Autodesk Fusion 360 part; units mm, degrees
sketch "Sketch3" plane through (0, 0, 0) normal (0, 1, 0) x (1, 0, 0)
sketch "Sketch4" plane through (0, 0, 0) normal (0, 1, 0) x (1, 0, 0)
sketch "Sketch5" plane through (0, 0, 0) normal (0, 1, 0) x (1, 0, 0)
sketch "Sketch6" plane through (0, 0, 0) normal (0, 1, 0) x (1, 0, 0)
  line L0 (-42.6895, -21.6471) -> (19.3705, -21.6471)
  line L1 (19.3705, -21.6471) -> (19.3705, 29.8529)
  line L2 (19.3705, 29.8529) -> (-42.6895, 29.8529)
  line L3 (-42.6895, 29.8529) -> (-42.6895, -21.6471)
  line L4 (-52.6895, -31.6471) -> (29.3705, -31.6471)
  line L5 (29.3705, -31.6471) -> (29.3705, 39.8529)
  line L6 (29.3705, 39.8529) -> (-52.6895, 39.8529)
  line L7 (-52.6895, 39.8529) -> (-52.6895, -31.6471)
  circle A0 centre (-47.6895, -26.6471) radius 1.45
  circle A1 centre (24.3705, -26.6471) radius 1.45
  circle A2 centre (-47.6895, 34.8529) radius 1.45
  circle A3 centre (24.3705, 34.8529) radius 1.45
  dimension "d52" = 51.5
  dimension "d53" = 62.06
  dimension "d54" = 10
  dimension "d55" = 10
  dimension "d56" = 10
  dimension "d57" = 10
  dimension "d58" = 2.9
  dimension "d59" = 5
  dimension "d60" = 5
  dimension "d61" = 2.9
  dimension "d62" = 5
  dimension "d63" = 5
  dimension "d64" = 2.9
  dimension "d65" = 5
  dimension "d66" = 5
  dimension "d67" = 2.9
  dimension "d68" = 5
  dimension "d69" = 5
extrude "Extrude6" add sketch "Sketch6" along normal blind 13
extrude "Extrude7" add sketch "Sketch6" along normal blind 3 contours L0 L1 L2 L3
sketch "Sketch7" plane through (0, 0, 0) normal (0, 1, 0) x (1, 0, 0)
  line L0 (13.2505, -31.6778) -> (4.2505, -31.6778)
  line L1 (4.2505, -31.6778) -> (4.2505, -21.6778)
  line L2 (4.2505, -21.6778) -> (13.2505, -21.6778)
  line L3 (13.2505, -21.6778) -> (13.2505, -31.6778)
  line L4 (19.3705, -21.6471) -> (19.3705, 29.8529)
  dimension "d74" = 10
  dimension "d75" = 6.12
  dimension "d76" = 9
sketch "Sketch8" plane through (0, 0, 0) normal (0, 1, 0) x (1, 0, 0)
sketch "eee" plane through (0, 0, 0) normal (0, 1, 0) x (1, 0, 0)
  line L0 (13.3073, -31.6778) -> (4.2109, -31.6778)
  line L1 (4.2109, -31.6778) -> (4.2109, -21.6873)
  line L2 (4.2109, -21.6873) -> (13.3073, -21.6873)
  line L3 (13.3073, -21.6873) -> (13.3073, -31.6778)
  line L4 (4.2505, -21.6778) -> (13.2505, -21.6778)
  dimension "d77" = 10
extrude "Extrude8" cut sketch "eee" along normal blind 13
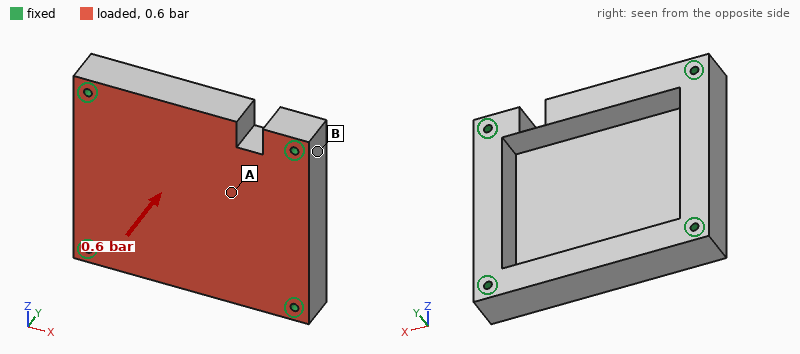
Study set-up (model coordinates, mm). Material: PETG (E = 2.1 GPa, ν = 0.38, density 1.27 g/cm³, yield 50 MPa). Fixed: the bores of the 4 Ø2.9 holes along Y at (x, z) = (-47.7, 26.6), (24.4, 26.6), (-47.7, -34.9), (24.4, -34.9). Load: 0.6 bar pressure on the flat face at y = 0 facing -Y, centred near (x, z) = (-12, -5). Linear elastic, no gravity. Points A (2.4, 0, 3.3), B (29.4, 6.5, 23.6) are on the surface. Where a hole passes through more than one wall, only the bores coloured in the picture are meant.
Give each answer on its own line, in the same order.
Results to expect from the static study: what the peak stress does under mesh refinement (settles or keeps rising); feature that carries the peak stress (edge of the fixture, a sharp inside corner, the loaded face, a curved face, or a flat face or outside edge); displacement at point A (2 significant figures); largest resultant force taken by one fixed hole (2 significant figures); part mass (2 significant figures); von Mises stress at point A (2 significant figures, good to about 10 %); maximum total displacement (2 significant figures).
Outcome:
keeps rising
a sharp inside corner
0.20 mm
110 N
54 g
3.0 MPa
0.26 mm
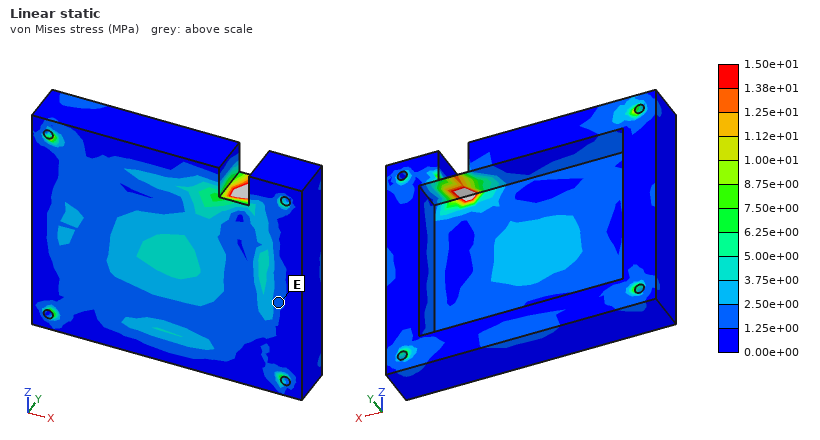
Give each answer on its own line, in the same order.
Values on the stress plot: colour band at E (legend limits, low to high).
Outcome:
1.25e+00 to 2.50e+00 MPa
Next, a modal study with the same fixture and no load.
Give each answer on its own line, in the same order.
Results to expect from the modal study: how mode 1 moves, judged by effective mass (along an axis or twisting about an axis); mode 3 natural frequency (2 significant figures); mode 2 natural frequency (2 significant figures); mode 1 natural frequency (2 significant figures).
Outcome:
along Y
2500 Hz
1700 Hz
1500 Hz
